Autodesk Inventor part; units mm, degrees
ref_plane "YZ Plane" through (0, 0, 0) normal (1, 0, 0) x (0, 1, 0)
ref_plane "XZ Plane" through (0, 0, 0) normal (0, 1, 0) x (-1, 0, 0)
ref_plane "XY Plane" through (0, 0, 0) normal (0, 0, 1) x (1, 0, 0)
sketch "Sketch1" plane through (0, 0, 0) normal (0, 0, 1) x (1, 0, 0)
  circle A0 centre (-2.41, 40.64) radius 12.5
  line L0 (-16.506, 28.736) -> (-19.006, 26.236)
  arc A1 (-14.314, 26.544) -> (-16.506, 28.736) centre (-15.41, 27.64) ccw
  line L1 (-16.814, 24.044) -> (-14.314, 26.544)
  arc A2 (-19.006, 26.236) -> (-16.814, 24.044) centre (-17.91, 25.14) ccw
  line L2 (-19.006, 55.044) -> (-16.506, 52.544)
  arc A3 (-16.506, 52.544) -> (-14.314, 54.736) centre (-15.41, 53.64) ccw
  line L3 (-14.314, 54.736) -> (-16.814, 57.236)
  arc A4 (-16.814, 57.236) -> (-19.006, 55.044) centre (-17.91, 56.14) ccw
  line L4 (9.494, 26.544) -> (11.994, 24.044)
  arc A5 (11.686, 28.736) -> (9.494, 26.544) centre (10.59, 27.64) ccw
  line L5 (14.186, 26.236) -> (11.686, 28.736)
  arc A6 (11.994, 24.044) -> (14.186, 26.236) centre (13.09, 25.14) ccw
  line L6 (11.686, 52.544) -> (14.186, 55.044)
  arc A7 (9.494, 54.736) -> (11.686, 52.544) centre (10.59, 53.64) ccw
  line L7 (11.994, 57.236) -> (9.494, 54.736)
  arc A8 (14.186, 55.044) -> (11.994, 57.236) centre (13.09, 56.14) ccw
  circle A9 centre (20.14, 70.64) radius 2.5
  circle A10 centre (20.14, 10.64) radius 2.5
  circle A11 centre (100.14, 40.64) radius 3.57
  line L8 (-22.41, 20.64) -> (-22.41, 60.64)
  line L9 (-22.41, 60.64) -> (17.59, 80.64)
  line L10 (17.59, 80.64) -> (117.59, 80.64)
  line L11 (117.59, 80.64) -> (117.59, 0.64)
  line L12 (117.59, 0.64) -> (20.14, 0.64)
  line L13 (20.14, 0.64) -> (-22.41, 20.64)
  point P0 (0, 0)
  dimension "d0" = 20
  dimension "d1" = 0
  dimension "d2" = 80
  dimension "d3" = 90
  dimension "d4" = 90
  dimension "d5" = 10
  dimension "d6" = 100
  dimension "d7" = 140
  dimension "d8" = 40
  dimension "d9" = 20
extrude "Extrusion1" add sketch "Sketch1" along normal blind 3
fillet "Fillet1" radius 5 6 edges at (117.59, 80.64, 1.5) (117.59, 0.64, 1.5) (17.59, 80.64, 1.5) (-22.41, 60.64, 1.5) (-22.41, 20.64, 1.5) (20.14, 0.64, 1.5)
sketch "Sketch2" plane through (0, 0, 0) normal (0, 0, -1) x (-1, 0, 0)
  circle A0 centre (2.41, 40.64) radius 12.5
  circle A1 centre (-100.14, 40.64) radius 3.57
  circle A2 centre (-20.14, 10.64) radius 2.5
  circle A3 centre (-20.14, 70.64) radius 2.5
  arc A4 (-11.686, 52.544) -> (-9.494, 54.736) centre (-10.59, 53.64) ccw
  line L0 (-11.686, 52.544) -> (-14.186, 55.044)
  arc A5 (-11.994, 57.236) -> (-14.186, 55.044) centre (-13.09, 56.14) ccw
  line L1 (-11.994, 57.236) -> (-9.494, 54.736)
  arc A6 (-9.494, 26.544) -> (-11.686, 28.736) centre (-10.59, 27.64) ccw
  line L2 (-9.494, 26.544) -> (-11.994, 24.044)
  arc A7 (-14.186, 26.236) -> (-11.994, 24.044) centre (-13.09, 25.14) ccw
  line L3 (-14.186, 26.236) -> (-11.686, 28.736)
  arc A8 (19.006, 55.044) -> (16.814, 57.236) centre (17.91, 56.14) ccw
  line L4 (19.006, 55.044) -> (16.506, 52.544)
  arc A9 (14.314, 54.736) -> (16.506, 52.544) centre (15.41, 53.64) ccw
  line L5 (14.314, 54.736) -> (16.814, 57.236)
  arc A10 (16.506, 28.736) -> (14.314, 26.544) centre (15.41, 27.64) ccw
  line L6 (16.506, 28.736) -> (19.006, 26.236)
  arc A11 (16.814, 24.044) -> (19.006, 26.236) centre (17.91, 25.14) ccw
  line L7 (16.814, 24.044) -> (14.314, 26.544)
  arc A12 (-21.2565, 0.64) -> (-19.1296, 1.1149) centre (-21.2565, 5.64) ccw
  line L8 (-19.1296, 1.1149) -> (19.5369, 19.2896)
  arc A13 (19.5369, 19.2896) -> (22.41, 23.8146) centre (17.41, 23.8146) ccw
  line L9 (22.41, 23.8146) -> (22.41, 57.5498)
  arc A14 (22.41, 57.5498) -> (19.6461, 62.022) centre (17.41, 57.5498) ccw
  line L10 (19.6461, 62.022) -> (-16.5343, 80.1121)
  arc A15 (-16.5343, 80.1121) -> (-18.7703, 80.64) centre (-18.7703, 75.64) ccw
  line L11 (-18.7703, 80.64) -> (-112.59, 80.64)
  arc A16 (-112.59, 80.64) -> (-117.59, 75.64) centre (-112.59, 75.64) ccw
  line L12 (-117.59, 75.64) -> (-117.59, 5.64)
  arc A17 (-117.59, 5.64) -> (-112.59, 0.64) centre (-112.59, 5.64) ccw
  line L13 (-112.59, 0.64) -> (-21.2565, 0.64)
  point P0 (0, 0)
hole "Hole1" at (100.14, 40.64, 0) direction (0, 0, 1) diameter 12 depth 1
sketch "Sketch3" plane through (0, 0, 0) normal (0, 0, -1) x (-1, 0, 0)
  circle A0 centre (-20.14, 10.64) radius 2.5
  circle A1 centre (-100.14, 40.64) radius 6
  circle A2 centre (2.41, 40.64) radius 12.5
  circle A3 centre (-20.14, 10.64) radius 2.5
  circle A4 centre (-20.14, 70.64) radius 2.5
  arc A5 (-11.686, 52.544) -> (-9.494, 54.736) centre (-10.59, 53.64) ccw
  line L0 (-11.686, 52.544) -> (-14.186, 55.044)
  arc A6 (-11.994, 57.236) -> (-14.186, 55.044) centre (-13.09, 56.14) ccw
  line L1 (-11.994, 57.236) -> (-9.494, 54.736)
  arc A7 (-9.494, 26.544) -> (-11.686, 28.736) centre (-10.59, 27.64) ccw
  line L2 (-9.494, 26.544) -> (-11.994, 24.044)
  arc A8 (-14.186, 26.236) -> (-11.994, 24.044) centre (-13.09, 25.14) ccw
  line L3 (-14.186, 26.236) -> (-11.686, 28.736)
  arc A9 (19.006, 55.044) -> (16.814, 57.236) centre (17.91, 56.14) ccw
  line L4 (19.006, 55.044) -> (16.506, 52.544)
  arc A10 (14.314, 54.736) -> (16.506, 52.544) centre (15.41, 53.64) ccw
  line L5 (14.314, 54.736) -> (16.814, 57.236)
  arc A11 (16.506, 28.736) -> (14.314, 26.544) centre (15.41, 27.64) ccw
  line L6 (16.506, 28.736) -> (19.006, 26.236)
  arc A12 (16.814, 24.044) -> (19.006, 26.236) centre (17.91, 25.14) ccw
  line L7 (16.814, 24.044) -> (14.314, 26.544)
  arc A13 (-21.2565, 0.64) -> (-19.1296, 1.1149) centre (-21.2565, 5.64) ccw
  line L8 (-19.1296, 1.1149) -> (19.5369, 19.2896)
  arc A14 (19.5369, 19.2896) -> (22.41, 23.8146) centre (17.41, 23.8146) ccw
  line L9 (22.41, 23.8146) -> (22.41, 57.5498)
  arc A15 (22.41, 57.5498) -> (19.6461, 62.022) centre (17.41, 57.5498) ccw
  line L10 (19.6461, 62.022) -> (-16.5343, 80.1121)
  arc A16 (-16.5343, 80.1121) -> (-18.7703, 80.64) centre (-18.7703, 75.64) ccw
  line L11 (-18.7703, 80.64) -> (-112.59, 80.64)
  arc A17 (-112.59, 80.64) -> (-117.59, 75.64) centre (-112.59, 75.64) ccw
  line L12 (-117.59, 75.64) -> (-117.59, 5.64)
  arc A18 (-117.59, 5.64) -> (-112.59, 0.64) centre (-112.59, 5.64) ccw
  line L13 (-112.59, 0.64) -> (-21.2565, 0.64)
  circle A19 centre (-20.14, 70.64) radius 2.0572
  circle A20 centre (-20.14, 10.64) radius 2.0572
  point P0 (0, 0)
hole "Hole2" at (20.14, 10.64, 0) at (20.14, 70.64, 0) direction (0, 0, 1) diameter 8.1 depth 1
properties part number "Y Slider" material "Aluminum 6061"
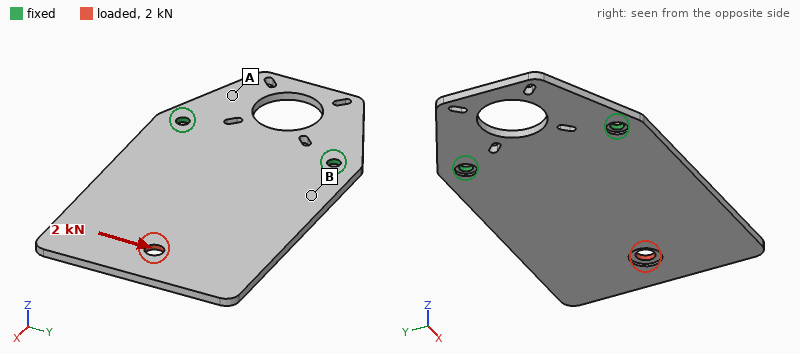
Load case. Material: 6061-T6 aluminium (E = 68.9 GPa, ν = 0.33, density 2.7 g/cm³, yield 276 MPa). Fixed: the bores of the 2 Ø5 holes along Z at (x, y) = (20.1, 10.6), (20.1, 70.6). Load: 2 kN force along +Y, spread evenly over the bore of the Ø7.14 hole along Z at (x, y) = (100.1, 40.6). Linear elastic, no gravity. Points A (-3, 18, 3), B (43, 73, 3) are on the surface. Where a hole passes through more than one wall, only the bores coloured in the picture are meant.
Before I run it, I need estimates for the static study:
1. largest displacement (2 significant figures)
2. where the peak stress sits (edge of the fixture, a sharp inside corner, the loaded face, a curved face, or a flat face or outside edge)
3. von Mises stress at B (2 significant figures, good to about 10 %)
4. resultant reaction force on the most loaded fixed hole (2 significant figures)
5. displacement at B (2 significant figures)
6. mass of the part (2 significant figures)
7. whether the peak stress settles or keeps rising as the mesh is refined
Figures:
0.20 mm
edge of the fixture
34 MPa
2.8 kN
0.045 mm
78 g
keeps rising
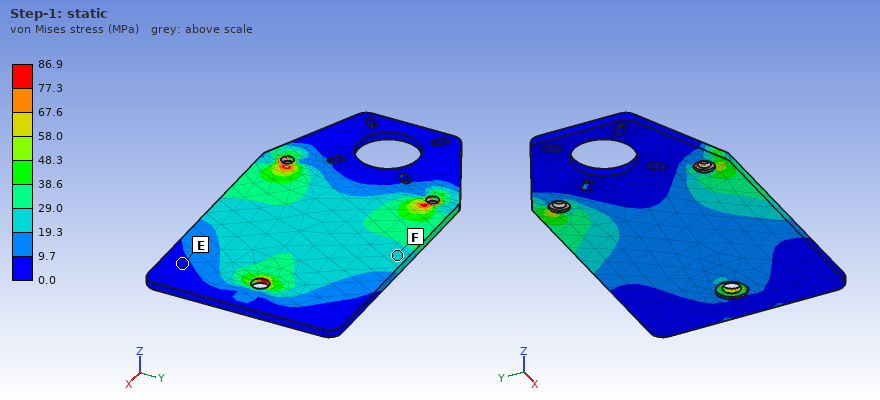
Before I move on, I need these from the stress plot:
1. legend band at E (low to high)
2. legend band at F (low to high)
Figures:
0.0 to 9.7 MPa
19.3 to 29.0 MPa
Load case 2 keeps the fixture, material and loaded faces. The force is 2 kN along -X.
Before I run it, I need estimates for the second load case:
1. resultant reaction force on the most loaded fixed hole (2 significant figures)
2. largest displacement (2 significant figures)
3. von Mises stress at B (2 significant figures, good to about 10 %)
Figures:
1.0 kN
0.37 mm
19 MPa
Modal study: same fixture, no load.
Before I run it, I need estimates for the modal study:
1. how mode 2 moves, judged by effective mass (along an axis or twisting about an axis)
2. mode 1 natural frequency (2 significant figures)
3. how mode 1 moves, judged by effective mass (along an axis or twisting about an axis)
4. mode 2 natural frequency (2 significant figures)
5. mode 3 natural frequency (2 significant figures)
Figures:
twisting about X
230 Hz
along Z
730 Hz
1300 Hz
